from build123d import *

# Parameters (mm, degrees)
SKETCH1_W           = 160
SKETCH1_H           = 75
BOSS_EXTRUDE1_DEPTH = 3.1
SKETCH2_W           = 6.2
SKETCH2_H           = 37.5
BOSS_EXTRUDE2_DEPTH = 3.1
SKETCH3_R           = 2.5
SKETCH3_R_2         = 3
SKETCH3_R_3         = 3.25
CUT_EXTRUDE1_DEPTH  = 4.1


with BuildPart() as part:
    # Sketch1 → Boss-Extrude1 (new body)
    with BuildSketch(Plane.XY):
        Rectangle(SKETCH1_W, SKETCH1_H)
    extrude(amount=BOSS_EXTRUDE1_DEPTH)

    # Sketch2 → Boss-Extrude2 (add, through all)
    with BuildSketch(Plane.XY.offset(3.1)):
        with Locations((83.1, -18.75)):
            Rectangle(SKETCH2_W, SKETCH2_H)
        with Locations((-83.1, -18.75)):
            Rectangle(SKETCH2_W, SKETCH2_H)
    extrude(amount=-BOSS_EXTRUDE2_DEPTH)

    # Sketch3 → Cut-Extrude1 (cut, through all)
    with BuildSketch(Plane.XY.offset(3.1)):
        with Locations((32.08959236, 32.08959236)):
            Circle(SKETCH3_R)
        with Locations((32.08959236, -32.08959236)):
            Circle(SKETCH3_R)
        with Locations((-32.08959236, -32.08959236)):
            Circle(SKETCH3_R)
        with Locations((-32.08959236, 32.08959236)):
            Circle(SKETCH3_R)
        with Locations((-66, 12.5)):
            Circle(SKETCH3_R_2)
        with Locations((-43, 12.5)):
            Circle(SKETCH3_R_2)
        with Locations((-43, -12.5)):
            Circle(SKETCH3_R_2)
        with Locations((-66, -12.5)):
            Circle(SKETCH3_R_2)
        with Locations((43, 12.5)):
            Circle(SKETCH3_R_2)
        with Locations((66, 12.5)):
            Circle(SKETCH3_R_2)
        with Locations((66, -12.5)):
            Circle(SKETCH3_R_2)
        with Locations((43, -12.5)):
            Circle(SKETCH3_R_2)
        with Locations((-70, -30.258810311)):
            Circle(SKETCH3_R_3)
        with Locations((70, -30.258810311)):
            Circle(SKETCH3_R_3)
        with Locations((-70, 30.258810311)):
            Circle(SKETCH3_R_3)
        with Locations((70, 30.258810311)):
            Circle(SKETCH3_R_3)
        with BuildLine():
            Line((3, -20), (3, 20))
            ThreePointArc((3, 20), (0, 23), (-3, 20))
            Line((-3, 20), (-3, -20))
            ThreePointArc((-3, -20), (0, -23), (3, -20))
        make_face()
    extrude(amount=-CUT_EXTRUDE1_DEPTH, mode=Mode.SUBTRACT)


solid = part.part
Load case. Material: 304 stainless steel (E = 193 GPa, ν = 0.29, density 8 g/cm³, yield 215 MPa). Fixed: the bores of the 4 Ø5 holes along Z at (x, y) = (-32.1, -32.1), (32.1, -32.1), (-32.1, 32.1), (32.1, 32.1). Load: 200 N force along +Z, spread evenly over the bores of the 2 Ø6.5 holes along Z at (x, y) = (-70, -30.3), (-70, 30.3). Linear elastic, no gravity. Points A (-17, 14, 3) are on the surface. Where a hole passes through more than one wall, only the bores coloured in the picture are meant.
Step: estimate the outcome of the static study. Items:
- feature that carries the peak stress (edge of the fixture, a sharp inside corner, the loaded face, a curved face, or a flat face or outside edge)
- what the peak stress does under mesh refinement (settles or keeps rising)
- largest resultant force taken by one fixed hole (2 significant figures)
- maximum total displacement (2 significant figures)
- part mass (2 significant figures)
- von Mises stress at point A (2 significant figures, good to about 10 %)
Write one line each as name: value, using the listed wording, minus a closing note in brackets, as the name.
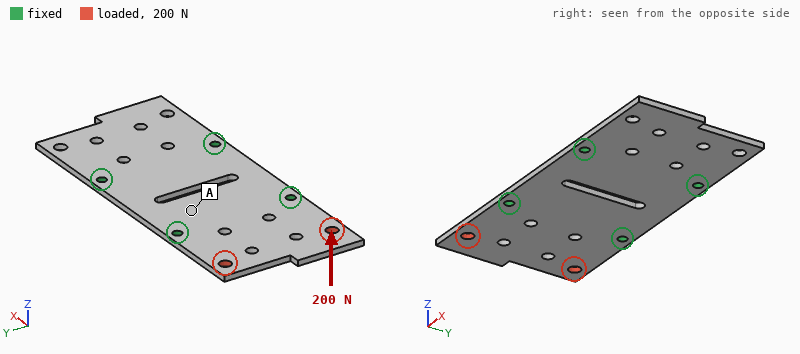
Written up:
feature that carries the peak stress: edge of the fixture
what the peak stress does under mesh refinement: keeps rising
largest resultant force taken by one fixed hole: 110 N
maximum total displacement: 0.21 mm
part mass: 290 g
von Mises stress at point A: 9.9 MPa
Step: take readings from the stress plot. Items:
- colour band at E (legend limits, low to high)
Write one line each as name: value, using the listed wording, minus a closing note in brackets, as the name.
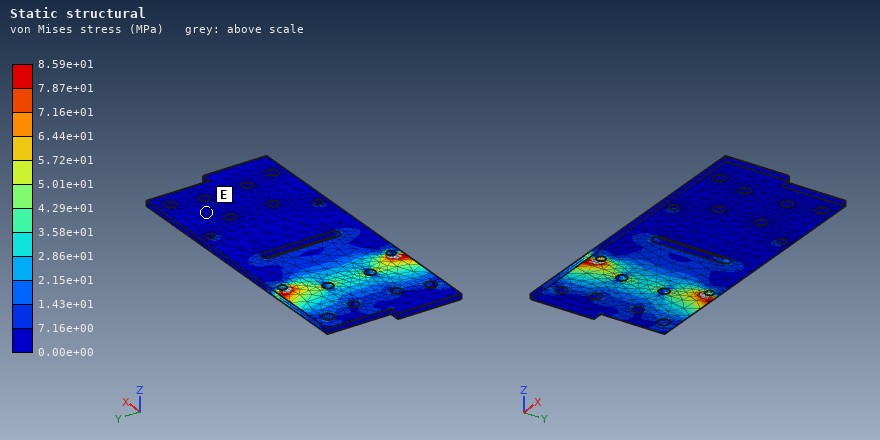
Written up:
colour band at E: 0.00e+00 to 7.16e+00 MPa
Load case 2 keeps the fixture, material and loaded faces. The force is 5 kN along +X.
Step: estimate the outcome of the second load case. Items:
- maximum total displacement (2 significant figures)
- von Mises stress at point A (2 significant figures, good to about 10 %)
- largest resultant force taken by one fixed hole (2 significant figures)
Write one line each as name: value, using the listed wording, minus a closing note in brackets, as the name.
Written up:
maximum total displacement: 11 µm
von Mises stress at point A: 9.5 MPa
largest resultant force taken by one fixed hole: 2.3 kN
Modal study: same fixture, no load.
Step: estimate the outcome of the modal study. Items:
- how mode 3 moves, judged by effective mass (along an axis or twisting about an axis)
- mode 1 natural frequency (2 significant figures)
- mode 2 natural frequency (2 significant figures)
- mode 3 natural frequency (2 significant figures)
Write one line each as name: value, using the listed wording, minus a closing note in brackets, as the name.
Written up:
how mode 3 moves, judged by effective mass: twisting about X
mode 1 natural frequency: 810 Hz
mode 2 natural frequency: 830 Hz
mode 3 natural frequency: 1800 Hz
